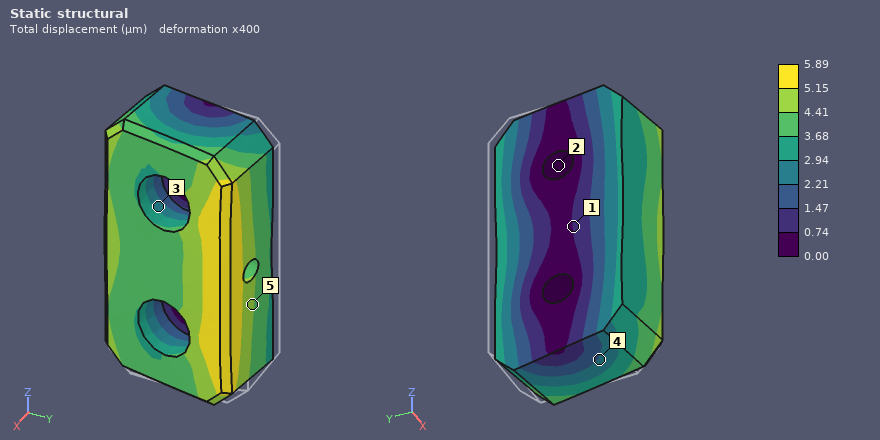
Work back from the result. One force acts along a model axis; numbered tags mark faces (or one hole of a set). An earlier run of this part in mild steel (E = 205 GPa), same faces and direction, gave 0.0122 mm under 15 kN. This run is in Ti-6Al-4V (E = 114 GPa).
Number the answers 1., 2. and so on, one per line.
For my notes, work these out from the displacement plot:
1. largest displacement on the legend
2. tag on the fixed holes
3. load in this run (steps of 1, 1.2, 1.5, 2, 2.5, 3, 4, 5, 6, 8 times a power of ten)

1. 5.89 µm
2. 2
3. 4 kN
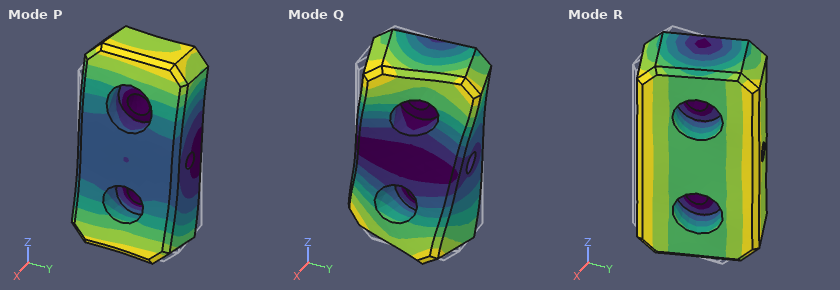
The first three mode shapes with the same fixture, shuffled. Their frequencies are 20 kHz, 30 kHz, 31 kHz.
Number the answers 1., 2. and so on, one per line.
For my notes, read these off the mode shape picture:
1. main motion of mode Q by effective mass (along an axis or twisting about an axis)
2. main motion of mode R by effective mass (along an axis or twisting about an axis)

1. twisting about X
2. along Y
